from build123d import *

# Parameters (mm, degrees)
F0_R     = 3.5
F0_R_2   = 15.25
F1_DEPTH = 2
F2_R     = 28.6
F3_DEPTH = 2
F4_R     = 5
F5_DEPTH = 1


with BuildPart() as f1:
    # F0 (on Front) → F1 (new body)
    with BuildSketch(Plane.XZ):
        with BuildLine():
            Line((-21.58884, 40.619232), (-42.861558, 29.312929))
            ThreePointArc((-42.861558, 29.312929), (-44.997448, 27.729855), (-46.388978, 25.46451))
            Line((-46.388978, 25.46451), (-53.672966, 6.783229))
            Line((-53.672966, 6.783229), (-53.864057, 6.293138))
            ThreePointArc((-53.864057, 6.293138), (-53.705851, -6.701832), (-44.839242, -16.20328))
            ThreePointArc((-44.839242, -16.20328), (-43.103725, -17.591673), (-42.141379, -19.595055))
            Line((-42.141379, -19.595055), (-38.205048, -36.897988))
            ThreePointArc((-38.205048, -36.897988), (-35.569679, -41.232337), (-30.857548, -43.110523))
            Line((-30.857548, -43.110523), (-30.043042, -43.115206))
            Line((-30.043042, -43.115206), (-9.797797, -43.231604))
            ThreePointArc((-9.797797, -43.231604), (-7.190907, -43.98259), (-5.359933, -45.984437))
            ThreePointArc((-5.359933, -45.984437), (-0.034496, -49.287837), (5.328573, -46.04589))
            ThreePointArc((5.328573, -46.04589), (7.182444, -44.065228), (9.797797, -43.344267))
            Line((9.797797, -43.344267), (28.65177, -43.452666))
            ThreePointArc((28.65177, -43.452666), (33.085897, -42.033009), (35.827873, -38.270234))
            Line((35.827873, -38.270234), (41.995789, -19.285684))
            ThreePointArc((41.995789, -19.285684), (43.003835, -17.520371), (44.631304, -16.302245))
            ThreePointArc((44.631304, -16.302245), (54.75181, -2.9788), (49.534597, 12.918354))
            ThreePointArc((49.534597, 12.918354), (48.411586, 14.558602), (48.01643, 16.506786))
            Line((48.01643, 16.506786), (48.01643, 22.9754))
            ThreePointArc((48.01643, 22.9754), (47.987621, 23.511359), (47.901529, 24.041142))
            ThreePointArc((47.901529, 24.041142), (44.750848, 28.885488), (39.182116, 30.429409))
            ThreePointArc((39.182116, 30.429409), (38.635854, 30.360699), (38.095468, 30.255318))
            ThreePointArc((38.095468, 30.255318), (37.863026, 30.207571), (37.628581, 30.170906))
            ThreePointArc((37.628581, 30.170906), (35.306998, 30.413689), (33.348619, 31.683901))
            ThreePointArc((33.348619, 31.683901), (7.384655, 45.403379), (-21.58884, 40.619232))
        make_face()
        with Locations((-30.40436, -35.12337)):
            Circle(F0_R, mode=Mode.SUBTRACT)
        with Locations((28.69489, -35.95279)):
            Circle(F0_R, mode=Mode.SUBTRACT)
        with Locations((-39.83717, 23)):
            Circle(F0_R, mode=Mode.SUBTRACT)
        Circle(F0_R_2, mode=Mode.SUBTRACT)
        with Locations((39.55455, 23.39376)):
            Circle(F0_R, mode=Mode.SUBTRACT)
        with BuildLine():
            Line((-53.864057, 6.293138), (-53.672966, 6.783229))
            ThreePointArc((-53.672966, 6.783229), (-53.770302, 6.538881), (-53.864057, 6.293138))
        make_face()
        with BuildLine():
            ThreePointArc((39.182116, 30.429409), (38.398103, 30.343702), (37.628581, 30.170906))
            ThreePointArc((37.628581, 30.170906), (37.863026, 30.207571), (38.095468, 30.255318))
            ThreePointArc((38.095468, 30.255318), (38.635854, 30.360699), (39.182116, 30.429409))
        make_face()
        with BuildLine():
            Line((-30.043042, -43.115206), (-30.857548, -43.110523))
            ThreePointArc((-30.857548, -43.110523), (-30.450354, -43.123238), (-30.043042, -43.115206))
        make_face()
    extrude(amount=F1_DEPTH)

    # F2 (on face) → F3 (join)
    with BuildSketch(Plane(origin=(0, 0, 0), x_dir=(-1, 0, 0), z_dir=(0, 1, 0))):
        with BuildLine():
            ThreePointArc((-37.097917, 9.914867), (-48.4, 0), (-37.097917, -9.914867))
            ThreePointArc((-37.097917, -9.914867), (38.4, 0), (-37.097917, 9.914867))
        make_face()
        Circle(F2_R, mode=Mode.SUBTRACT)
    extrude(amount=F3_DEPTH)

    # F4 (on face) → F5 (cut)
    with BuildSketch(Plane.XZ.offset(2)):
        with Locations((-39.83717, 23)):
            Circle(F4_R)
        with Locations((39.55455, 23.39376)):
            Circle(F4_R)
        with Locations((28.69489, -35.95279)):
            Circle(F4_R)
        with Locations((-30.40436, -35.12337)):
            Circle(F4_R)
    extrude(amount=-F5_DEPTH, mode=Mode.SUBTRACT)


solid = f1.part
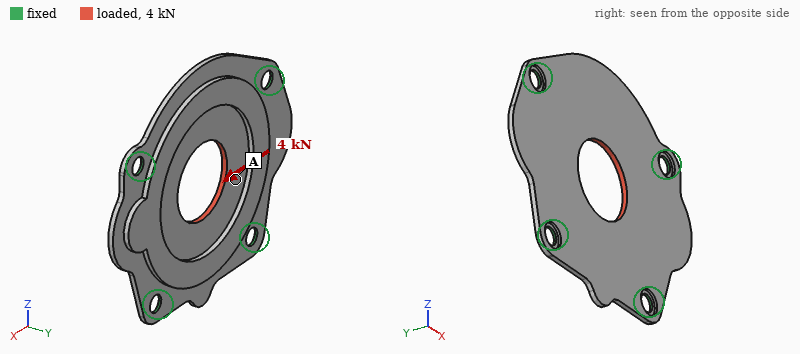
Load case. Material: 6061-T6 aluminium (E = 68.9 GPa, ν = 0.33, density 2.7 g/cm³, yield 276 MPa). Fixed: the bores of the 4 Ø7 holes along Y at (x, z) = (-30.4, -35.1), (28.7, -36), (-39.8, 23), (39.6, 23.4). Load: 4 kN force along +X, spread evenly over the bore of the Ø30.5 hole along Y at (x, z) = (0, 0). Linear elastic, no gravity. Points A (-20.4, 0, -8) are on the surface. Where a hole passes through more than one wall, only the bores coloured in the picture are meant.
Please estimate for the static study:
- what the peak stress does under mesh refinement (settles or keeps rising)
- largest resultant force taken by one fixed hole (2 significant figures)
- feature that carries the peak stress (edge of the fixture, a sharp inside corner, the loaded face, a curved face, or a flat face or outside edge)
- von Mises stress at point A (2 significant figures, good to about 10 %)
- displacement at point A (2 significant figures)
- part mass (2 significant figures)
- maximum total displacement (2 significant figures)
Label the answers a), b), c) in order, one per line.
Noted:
a) keeps rising
b) 1.1 kN
c) edge of the fixture
d) 18 MPa
e) 14 µm
f) 48 g
g) 19 µm
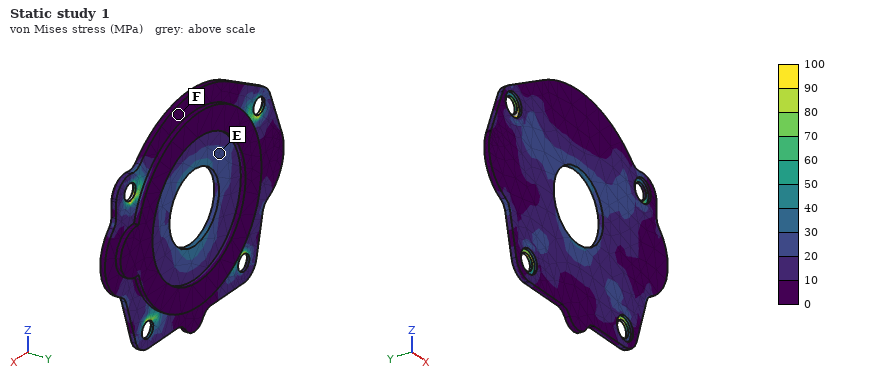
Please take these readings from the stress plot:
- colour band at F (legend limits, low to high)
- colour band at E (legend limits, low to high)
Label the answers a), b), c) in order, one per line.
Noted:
a) 0 to 10 MPa
b) 20 to 30 MPa
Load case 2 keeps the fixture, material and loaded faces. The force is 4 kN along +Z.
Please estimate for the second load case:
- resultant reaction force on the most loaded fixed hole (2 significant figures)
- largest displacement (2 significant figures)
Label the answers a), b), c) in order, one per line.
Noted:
a) 1.1 kN
b) 35 µm
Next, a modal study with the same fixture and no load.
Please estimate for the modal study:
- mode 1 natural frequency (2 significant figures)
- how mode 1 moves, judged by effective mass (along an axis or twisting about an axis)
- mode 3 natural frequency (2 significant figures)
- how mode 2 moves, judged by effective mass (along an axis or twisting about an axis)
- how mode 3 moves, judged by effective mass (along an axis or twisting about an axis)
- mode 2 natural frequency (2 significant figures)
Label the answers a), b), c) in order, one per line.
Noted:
a) 1800 Hz
b) along Y
c) 3200 Hz
d) along Y
e) twisting about Z
f) 2600 Hz
